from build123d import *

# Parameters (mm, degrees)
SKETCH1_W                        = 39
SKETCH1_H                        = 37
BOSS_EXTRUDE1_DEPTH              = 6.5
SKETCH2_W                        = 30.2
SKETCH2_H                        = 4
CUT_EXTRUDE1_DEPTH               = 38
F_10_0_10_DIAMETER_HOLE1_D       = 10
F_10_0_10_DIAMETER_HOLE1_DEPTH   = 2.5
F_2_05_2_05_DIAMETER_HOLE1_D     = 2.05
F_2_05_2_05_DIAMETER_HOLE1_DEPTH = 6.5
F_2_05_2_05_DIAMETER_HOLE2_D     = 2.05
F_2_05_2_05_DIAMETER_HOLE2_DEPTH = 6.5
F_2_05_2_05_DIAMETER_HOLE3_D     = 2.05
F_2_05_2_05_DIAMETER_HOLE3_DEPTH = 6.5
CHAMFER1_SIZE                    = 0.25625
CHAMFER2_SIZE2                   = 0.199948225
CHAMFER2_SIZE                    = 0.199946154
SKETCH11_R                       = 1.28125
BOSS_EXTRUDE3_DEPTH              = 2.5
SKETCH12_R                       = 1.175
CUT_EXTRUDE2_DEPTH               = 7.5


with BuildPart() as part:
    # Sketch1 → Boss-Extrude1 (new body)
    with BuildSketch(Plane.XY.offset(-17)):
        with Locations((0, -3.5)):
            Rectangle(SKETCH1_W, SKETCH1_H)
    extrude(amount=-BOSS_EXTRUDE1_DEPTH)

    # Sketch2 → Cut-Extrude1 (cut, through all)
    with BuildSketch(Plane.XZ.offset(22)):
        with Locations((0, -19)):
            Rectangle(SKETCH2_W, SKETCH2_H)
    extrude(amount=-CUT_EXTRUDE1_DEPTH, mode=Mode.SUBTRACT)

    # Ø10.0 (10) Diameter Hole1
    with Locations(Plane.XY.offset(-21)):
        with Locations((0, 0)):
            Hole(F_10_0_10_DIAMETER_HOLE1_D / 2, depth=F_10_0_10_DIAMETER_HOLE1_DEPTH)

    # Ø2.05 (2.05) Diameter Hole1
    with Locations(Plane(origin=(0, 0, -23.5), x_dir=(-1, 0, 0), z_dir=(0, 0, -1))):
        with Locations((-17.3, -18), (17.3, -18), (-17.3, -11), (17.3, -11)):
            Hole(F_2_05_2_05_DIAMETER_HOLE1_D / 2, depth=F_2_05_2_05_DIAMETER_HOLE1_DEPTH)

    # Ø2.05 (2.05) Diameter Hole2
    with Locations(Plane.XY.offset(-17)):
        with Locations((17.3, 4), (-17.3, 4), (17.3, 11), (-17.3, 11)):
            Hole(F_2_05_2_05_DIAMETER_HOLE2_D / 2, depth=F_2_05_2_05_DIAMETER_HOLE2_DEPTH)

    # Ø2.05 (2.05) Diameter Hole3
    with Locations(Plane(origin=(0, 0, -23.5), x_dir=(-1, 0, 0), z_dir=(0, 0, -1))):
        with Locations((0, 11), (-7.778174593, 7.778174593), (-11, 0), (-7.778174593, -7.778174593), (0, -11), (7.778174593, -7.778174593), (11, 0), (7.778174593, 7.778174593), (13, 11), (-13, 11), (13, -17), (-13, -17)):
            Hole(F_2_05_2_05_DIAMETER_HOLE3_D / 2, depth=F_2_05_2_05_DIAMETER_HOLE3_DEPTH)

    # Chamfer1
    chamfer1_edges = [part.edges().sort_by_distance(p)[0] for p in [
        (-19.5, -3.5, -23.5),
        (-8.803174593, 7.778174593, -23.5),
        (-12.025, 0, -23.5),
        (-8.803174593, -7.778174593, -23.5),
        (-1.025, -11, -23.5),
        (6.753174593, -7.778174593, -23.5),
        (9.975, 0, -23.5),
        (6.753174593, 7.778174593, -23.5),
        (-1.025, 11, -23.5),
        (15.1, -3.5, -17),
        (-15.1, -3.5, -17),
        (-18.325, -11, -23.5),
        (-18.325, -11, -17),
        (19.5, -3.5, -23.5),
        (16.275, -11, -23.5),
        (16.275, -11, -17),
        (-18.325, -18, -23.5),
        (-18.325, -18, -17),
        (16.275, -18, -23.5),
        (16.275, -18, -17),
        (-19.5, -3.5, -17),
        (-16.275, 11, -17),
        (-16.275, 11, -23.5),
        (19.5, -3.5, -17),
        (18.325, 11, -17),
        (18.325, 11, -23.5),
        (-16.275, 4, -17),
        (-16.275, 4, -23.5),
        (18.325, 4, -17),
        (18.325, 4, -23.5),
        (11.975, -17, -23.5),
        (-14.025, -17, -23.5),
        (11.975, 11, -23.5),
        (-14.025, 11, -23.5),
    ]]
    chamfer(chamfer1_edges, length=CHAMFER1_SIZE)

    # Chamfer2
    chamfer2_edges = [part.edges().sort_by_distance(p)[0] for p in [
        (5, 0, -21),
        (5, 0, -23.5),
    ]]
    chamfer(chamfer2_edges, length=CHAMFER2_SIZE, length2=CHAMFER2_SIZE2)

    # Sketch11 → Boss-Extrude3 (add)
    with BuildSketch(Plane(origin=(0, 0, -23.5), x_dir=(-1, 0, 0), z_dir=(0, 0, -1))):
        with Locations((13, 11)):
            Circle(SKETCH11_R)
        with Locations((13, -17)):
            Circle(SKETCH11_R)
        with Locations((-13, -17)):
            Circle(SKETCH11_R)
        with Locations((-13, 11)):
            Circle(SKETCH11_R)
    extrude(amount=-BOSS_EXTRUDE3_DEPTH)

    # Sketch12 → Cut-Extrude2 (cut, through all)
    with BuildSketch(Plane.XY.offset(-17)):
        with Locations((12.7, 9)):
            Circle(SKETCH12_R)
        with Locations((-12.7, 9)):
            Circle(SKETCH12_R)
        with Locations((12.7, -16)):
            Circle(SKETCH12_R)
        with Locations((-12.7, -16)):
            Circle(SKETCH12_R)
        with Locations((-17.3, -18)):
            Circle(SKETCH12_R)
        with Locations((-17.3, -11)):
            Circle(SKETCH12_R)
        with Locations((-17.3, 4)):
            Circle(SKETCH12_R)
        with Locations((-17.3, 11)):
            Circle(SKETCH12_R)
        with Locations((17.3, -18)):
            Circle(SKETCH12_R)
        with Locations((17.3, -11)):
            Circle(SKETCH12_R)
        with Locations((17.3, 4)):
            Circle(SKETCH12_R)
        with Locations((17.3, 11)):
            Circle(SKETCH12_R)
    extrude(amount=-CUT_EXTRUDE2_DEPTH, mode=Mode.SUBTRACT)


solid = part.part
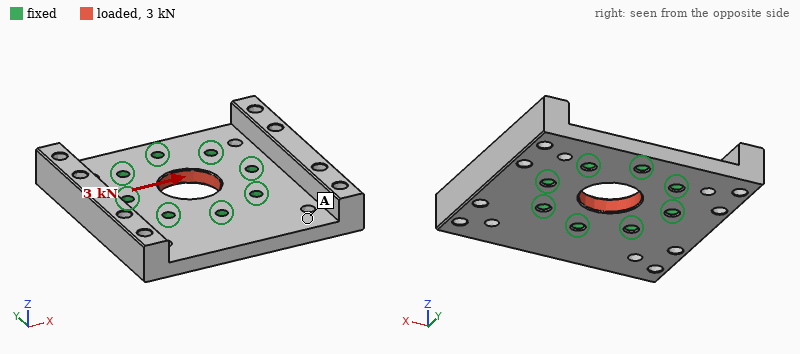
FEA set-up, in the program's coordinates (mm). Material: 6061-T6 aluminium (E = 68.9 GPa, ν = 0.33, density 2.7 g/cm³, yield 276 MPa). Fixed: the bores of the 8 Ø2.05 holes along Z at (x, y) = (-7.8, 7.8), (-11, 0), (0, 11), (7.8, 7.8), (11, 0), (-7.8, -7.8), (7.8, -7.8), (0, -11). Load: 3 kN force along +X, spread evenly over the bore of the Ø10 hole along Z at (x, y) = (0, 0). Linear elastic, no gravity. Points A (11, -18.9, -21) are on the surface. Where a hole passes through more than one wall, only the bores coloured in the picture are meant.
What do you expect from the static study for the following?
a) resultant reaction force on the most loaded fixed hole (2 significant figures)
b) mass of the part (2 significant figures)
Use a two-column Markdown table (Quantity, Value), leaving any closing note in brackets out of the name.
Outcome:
| Quantity | Value |
|---|---|
| resultant reaction force on the most loaded fixed hole | 580 N |
| mass of the part | 12 g |
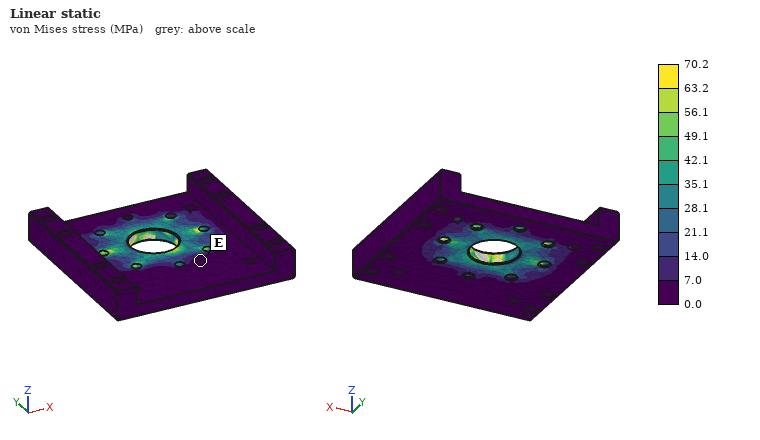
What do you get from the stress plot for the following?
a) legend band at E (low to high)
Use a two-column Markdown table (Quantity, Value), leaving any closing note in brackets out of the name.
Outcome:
| Quantity | Value |
|---|---|
| legend band at E | 0.0 to 7.0 MPa |
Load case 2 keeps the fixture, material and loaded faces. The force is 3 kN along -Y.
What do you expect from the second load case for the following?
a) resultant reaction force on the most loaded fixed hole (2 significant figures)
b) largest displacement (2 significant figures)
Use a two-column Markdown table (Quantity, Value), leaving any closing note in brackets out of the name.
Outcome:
| Quantity | Value |
|---|---|
| resultant reaction force on the most loaded fixed hole | 580 N |
| largest displacement | 3.9 µm |
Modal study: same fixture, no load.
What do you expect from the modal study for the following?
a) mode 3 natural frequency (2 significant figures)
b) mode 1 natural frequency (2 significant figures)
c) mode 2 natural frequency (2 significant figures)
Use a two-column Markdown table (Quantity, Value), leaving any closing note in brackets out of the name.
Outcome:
| Quantity | Value |
|---|---|
| mode 3 natural frequency | 12 kHz |
| mode 1 natural frequency | 8600 Hz |
| mode 2 natural frequency | 8800 Hz |
